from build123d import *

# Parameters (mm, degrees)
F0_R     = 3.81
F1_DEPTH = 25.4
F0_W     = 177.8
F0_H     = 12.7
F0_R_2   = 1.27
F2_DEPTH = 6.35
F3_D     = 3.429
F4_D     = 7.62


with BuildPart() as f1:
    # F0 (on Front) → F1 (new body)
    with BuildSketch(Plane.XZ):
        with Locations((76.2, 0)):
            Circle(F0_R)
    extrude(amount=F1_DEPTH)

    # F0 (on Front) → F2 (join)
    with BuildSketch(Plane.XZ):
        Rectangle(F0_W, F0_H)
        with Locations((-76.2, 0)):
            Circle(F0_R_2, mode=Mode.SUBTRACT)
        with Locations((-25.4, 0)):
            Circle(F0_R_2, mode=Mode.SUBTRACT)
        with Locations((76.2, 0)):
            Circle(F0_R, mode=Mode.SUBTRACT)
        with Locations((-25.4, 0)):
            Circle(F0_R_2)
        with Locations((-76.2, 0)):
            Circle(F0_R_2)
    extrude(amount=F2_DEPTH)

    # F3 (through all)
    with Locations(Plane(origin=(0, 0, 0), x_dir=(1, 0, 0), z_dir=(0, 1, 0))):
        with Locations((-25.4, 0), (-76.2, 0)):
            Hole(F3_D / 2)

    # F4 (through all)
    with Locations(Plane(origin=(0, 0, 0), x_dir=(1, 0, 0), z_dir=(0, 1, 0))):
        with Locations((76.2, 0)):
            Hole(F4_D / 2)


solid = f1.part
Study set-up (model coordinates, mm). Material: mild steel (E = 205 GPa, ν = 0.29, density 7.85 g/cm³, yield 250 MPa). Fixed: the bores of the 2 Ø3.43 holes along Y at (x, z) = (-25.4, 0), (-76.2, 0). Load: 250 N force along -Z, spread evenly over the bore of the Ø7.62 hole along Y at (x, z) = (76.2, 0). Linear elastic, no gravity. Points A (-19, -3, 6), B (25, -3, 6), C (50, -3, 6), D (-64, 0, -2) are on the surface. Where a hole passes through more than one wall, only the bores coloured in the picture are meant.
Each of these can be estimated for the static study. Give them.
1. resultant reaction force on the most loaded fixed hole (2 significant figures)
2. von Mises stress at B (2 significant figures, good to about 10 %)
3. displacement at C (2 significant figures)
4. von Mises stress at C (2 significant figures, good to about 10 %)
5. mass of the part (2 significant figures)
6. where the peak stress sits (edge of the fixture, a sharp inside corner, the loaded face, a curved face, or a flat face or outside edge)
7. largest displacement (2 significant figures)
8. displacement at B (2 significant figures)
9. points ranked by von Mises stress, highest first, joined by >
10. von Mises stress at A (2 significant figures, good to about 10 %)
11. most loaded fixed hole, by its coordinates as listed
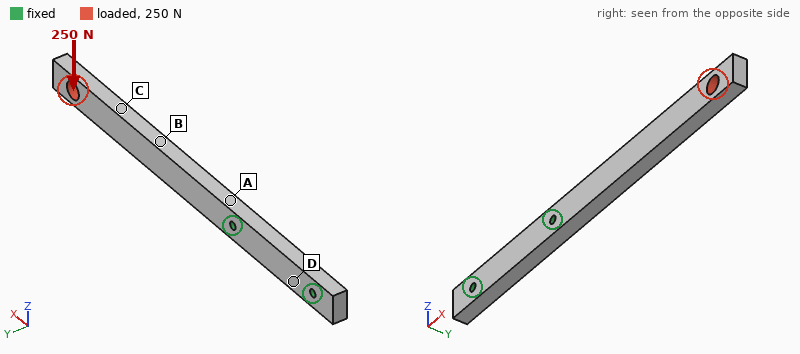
500 N
75 MPa
0.30 mm
39 MPa
110 g
edge of the fixture
0.55 mm
0.16 mm
A > B > C > D
140 MPa
(-25.4, 0)
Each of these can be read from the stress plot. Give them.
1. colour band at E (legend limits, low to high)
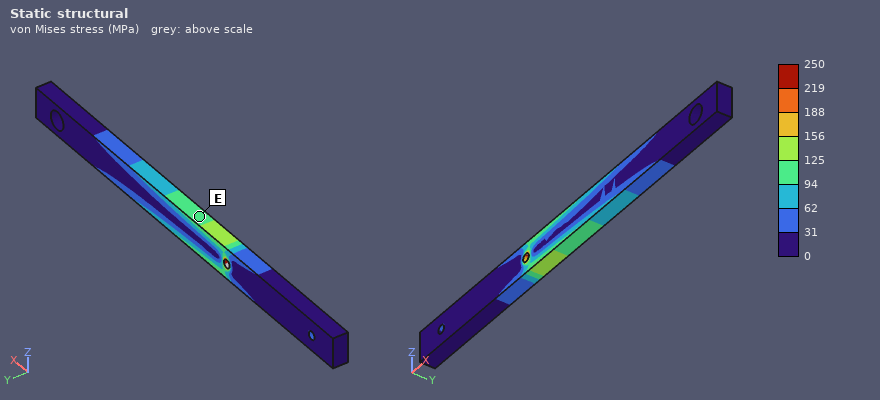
94 to 125 MPa
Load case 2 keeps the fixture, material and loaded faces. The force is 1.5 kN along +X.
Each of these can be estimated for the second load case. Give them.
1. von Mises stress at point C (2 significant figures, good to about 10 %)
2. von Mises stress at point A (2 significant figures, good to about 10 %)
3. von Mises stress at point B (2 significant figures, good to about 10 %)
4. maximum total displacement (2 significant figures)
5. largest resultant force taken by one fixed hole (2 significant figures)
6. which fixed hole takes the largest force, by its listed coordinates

19 MPa
14 MPa
19 MPa
10 µm
1.4 kN
(-25.4, 0)
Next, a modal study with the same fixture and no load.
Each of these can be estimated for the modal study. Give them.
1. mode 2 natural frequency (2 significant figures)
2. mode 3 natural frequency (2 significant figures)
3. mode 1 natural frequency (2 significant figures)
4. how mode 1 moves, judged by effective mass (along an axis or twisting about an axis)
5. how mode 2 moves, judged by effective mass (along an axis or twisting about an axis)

760 Hz
2500 Hz
420 Hz
along Y
along Z
